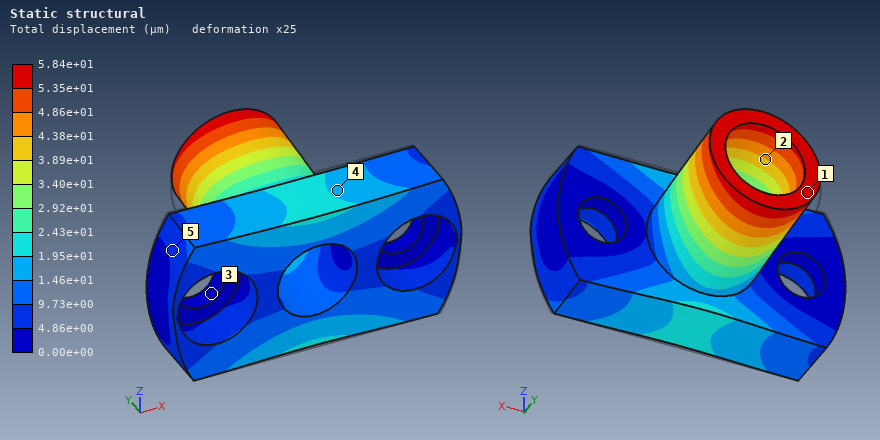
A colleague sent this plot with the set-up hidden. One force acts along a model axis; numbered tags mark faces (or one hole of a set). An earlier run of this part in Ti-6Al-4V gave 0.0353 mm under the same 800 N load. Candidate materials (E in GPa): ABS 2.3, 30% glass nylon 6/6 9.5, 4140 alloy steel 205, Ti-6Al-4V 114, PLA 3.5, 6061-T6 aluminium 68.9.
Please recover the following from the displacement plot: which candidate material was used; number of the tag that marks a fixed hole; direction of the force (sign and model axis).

6061-T6 aluminium
3
+Z
